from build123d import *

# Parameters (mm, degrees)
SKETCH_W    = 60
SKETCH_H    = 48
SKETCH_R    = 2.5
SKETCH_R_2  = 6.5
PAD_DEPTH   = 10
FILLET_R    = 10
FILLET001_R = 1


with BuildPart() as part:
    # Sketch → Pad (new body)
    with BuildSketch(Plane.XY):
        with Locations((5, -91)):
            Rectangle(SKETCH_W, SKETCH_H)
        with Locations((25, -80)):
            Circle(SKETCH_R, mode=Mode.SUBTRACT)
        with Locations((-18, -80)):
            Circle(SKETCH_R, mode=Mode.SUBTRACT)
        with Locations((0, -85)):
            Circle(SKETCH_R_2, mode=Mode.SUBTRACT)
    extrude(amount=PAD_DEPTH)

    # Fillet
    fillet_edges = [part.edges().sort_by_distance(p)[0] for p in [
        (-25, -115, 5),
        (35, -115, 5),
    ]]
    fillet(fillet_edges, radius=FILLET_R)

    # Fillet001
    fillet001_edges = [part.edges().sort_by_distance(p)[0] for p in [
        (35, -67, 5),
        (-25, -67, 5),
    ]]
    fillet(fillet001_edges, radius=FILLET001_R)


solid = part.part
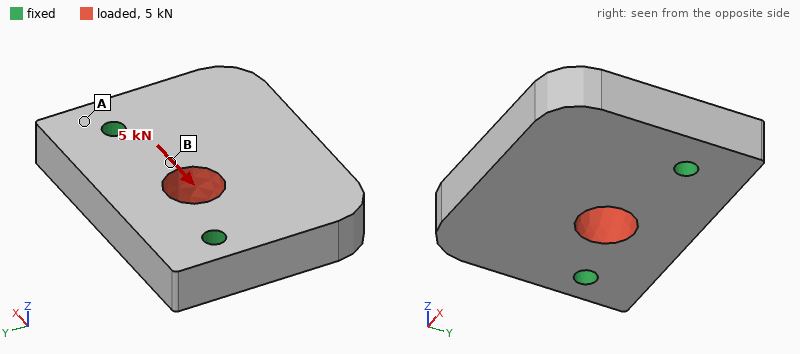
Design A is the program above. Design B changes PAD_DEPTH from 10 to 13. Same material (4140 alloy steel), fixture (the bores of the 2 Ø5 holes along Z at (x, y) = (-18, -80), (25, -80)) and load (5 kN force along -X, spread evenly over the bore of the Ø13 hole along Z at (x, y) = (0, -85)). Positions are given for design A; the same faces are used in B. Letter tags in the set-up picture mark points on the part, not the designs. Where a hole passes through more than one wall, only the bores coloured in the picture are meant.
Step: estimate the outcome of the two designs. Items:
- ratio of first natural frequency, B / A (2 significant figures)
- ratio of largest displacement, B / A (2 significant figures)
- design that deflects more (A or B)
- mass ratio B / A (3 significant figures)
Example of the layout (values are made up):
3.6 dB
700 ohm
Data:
1.2
0.77
A
1.30
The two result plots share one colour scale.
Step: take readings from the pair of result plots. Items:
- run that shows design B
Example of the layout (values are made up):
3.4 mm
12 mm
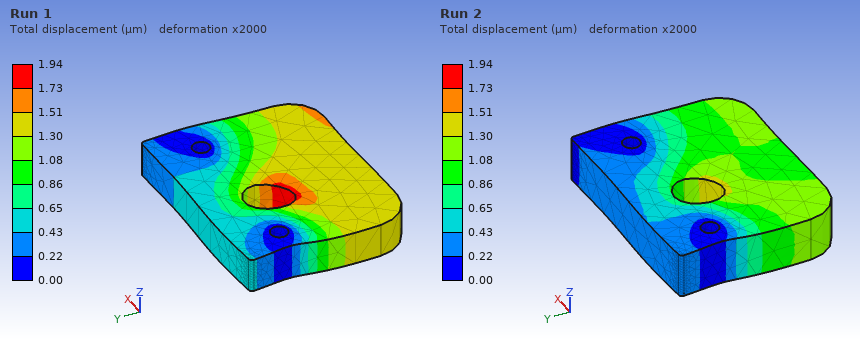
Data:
Run 2
